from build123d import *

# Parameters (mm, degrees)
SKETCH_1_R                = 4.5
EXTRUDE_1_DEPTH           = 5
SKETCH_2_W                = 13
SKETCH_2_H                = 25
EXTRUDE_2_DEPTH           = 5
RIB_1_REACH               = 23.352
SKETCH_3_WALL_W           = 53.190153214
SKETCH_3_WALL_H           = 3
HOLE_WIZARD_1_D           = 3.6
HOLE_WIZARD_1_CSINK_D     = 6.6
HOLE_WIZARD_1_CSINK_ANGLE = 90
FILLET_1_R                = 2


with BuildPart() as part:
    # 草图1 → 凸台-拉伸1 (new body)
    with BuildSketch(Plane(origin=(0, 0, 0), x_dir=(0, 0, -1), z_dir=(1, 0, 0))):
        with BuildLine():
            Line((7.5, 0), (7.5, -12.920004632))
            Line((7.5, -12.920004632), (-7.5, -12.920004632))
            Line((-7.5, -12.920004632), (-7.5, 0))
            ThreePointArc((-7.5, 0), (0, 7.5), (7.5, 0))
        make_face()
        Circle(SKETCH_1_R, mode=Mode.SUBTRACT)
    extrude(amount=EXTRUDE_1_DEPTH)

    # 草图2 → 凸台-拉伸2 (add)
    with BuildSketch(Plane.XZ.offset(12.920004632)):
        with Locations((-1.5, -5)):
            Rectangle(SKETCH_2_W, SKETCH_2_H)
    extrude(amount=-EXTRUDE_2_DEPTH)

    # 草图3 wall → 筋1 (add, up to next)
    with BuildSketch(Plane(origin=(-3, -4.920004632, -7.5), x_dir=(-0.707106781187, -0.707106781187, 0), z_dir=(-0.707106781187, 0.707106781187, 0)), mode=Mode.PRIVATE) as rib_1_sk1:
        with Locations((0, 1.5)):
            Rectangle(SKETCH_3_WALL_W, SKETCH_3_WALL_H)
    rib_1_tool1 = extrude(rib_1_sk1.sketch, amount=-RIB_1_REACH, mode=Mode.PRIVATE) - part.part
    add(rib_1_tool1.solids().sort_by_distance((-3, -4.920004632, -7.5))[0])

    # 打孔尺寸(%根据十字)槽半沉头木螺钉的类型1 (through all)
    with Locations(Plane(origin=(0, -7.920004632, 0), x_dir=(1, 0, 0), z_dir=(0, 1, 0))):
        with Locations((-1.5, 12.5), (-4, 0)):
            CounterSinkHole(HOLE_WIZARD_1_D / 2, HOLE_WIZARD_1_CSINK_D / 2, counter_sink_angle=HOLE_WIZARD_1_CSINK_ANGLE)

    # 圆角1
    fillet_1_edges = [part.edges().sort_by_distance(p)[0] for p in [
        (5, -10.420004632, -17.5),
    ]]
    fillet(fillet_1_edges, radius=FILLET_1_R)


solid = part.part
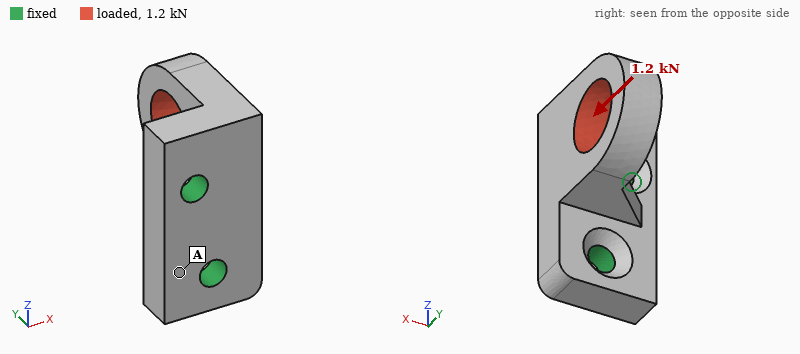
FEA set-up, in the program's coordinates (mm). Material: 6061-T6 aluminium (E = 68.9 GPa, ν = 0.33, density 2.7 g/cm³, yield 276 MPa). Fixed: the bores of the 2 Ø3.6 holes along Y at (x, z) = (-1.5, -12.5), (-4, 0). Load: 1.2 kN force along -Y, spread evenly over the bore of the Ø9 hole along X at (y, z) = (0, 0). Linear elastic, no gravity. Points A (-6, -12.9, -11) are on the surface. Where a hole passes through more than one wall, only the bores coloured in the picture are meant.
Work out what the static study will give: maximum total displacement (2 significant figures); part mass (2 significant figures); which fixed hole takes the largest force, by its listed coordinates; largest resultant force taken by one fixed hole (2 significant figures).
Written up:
54 µm
6.1 g
(-4, 0)
990 N
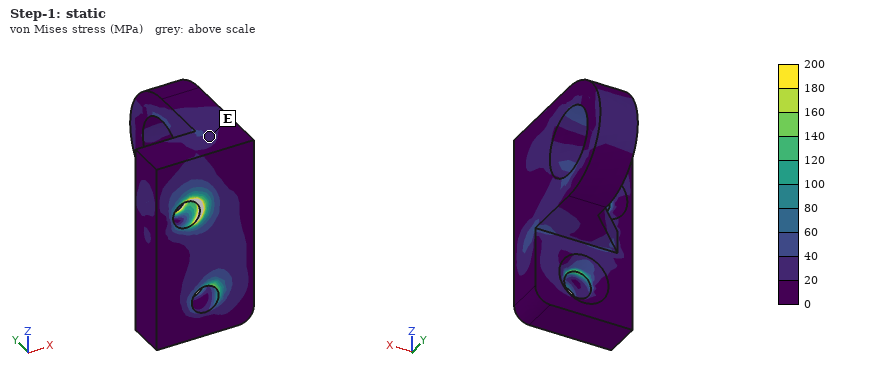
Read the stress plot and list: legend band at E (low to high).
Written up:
20 to 40 MPa
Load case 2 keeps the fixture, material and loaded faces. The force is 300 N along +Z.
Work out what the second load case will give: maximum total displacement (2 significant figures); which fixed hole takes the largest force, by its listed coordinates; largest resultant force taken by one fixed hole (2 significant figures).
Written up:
20 µm
(-1.5, -12.5)
310 N
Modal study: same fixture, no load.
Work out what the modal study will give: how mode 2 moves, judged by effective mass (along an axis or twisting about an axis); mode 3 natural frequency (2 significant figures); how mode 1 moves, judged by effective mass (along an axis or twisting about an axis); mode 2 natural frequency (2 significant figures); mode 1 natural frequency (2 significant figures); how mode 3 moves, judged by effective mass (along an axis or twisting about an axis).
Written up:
along Z
30 kHz
along X
17 kHz
12 kHz
along Y
